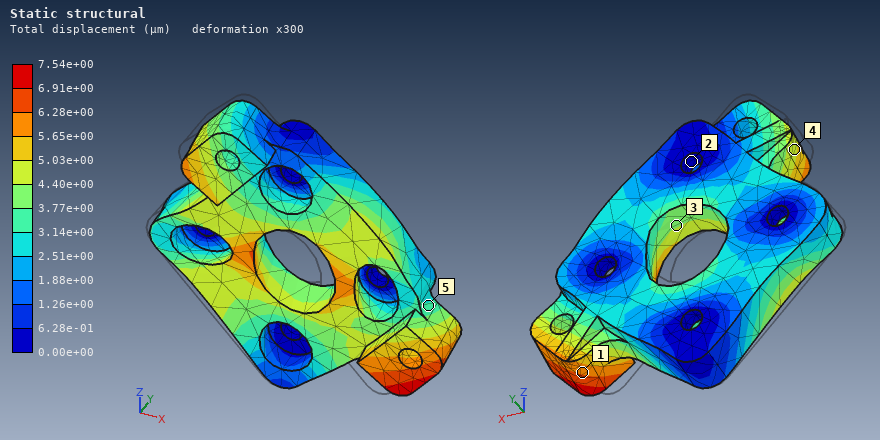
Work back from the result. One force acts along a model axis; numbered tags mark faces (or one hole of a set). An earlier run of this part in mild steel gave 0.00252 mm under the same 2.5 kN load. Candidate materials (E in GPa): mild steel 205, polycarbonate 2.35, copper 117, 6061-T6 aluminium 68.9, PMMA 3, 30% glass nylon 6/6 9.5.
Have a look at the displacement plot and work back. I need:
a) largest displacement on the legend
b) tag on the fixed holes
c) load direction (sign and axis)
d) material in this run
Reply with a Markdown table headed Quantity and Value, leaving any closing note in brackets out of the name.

| Quantity | Value |
|---|---|
| largest displacement on the legend | 7.54e+00 µm |
| tag on the fixed holes | 2 |
| load direction | +X |
| material in this run | 6061-T6 aluminium |
